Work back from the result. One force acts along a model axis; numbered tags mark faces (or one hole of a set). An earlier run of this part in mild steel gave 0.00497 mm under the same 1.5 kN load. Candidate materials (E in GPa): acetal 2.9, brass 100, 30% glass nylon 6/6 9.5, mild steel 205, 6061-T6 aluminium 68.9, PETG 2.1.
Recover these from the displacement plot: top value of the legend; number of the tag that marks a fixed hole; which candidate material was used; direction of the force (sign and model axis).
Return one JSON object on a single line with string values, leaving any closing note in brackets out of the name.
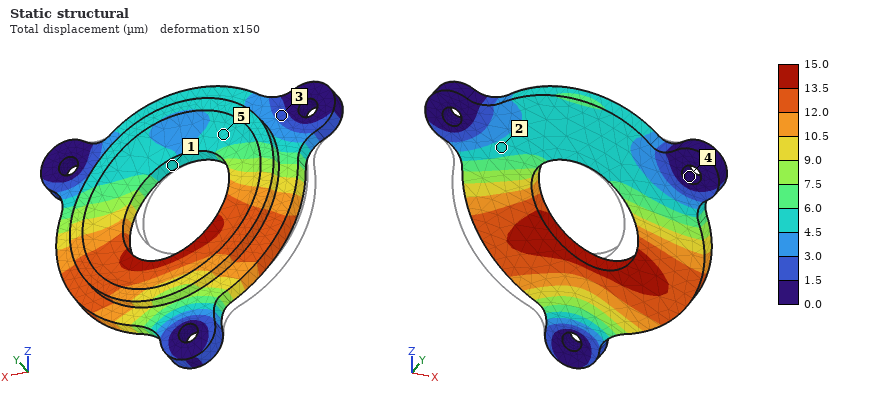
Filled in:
{"top value of the legend": "15.0 µm", "number of the tag that marks a fixed hole": "4", "which candidate material was used": "6061-T6 aluminium", "direction of the force": "+X"}
